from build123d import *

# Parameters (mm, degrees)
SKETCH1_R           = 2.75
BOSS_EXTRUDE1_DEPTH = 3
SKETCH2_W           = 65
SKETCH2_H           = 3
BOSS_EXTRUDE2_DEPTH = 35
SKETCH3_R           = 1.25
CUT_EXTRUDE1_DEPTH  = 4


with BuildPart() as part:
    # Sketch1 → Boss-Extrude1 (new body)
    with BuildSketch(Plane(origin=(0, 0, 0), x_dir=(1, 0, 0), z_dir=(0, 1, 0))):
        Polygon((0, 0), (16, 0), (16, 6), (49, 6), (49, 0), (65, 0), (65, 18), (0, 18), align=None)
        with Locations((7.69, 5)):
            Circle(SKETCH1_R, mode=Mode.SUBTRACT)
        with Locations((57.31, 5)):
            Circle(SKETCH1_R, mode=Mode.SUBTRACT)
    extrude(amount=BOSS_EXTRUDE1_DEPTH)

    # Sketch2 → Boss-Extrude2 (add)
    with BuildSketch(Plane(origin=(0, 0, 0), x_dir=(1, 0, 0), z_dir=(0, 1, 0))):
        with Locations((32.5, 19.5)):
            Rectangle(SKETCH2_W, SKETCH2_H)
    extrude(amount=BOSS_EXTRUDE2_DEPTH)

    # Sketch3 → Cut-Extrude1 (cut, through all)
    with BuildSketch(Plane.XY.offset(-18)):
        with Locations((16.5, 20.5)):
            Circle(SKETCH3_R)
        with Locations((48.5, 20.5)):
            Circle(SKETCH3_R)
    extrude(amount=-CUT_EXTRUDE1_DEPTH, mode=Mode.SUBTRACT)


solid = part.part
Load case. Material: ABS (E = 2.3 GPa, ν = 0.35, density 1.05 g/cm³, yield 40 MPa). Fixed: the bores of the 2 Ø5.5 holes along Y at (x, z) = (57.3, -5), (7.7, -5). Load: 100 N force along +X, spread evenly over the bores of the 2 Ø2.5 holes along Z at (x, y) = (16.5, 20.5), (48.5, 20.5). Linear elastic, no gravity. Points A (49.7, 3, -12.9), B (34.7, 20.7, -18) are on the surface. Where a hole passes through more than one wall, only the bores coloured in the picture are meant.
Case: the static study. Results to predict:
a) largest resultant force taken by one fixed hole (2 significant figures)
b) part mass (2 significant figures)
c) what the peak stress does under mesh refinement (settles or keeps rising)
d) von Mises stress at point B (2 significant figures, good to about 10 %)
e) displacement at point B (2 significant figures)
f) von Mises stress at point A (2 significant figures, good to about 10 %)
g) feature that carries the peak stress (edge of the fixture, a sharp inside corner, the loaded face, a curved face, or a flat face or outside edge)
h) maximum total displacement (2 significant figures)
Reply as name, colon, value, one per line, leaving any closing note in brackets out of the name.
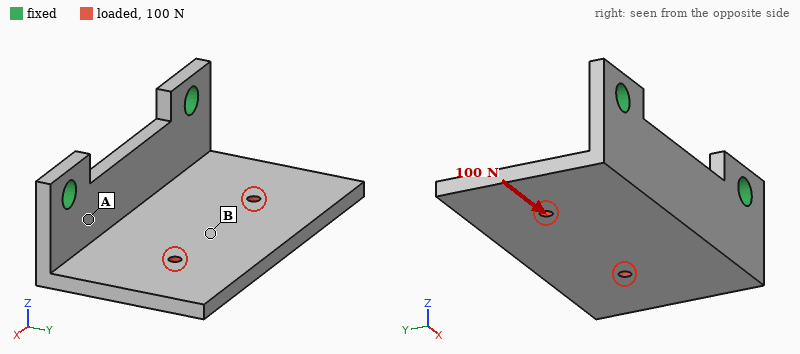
largest resultant force taken by one fixed hole: 66 N
part mass: 10 g
what the peak stress does under mesh refinement: keeps rising
von Mises stress at point B: 1.7 MPa
displacement at point B: 0.18 mm
von Mises stress at point A: 4.3 MPa
feature that carries the peak stress: edge of the fixture
maximum total displacement: 0.49 mm
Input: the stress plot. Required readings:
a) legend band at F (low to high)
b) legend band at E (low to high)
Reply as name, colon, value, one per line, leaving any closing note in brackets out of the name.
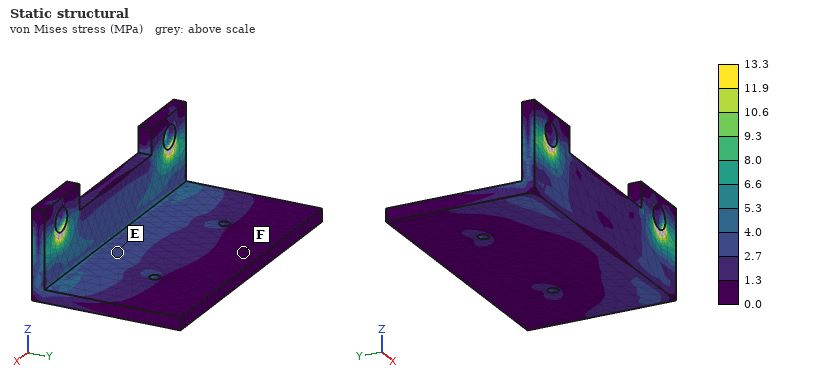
legend band at F: 0.0 to 1.3 MPa
legend band at E: 2.7 to 4.0 MPa
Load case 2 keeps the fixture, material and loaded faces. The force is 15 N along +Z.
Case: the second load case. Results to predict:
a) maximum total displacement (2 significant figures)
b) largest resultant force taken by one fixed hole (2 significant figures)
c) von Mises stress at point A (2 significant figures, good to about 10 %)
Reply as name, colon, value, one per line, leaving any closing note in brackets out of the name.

maximum total displacement: 0.71 mm
largest resultant force taken by one fixed hole: 8.7 N
von Mises stress at point A: 3.4 MPa
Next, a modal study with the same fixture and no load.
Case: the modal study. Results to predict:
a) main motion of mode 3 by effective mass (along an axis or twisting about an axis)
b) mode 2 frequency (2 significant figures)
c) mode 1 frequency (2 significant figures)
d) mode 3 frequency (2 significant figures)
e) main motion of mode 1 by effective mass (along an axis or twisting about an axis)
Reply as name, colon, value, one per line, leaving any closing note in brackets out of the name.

main motion of mode 3 by effective mass: along Y
mode 2 frequency: 750 Hz
mode 1 frequency: 350 Hz
mode 3 frequency: 1300 Hz
main motion of mode 1 by effective mass: along Z
